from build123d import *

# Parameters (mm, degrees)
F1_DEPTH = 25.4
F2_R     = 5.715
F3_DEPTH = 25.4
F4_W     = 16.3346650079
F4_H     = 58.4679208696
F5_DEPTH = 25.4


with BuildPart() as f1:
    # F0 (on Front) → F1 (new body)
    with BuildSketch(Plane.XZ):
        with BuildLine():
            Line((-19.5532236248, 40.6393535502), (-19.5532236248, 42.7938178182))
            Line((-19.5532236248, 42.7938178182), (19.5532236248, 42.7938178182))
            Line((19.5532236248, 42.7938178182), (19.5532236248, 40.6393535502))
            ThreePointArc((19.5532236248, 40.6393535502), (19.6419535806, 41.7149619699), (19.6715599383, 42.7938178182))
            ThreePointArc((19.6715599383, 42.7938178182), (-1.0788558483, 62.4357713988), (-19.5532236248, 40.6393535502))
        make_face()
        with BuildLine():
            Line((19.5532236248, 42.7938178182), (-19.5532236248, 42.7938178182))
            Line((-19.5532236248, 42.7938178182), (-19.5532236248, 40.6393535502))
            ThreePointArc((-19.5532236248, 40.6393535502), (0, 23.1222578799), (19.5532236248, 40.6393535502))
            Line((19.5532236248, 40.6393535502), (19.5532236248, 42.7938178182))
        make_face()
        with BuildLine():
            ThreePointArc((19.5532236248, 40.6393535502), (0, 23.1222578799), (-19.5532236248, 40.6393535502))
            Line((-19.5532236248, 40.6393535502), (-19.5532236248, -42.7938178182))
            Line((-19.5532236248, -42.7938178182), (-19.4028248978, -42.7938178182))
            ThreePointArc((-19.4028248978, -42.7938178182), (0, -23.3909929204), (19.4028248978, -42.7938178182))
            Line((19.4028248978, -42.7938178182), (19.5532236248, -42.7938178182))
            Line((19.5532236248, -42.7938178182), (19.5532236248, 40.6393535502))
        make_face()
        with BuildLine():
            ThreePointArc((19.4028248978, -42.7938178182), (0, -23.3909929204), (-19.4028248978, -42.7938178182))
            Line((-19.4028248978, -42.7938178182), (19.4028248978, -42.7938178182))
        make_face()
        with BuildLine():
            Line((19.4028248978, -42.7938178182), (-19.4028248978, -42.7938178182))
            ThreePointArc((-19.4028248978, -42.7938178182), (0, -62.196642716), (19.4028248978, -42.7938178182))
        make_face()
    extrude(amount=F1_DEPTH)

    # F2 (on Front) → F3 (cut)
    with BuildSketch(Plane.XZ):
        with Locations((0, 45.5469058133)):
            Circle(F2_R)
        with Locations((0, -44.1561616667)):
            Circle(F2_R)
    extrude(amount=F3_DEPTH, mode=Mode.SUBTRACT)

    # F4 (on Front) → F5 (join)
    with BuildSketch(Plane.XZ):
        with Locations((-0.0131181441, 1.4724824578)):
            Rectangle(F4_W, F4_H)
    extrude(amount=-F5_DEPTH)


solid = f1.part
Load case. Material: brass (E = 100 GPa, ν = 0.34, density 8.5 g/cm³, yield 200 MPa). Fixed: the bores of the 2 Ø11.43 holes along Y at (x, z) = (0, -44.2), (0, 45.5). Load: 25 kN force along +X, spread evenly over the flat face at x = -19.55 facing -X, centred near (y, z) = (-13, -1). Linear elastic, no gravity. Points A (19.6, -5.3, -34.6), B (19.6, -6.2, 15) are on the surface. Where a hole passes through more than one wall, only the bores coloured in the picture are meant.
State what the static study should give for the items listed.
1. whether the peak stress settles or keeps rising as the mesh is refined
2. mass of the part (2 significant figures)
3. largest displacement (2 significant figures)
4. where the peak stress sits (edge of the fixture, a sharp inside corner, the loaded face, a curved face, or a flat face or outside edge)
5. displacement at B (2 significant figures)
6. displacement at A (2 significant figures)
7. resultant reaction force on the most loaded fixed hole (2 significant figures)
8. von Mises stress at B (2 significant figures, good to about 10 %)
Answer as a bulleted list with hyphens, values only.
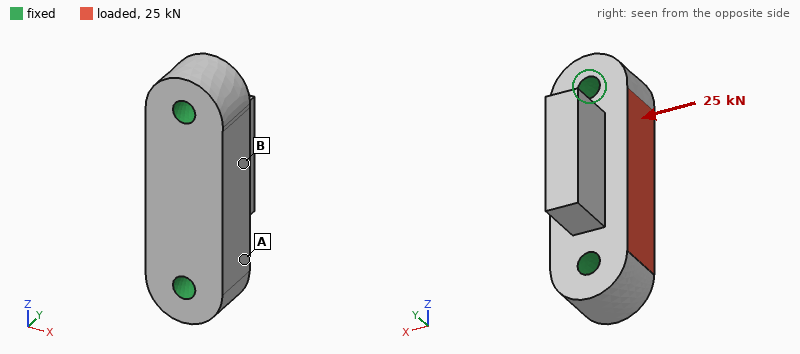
- keeps rising
- 1.1 kg
- 18 µm
- edge of the fixture
- 13 µm
- 7.1 µm
- 13 kN
- 21 MPa
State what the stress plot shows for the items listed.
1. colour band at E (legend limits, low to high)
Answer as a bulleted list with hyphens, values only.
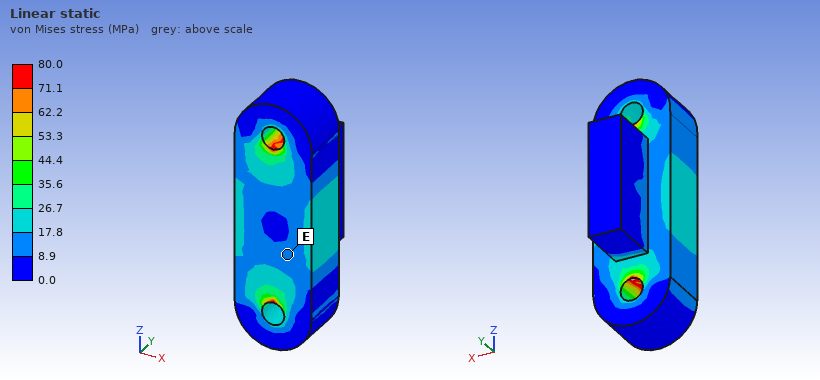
- 8.9 to 17.8 MPa
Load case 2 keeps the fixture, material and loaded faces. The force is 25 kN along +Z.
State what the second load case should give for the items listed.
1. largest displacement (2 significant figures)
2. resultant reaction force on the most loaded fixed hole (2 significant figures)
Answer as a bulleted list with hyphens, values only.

- 7.6 µm
- 14 kN
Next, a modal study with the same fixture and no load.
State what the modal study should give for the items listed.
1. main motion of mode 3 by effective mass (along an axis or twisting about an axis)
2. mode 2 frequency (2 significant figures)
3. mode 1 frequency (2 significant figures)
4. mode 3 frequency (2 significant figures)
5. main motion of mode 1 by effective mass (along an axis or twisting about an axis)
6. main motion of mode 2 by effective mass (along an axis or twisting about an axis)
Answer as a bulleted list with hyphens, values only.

- along X
- 7500 Hz
- 5100 Hz
- 8300 Hz
- along X
- along Y
